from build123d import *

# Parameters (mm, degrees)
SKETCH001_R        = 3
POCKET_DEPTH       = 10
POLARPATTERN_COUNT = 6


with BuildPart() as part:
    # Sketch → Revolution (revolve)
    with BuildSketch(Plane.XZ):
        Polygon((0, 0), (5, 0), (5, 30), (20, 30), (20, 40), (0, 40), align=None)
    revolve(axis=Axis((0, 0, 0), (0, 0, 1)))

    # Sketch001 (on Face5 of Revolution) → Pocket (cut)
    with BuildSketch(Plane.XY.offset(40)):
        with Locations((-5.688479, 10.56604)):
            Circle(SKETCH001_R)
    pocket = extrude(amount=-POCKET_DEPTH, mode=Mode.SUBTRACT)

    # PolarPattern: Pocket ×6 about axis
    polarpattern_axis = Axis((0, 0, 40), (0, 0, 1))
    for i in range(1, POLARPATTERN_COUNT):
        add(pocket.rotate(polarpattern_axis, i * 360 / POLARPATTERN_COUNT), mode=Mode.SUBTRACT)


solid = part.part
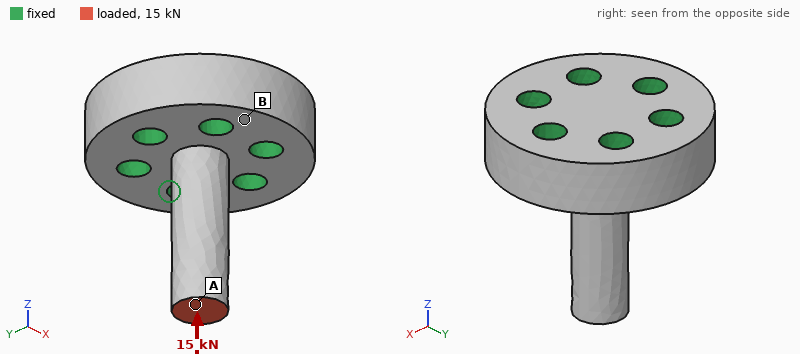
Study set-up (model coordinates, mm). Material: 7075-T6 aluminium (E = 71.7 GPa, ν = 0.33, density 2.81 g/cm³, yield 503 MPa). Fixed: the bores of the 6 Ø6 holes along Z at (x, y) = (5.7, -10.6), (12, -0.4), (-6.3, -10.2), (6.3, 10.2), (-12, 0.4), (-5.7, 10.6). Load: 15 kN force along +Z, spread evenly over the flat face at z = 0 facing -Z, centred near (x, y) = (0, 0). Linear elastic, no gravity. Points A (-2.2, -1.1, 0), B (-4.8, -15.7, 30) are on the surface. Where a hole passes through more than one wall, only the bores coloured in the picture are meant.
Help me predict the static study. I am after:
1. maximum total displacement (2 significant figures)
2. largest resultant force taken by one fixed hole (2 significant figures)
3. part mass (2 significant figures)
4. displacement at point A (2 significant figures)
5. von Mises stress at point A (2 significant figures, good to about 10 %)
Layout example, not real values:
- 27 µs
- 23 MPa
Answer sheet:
- 93 µm
- 2.9 kN
- 37 g
- 93 µm
- 190 MPa
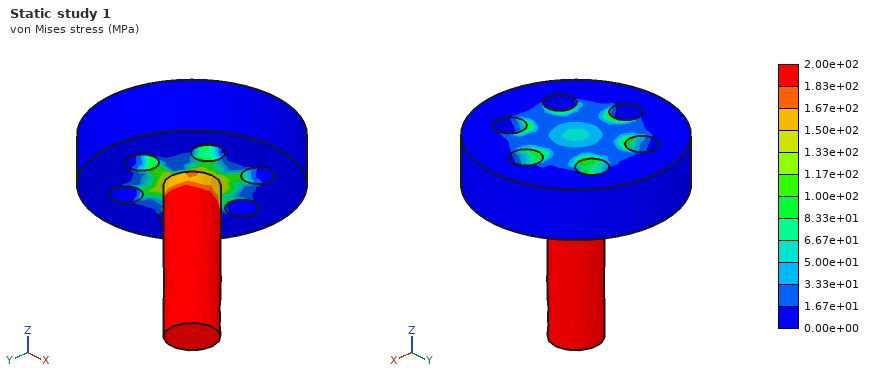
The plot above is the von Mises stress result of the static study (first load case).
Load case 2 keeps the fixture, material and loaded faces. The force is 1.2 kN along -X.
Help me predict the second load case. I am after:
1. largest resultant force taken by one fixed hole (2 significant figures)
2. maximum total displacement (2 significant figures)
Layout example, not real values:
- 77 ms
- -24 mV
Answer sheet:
- 1.5 kN
- 0.40 mm
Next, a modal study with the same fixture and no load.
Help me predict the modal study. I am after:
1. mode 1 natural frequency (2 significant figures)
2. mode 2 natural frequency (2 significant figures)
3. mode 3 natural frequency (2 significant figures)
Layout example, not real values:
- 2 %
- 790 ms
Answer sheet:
- 6600 Hz
- 6600 Hz
- 25 kHz
